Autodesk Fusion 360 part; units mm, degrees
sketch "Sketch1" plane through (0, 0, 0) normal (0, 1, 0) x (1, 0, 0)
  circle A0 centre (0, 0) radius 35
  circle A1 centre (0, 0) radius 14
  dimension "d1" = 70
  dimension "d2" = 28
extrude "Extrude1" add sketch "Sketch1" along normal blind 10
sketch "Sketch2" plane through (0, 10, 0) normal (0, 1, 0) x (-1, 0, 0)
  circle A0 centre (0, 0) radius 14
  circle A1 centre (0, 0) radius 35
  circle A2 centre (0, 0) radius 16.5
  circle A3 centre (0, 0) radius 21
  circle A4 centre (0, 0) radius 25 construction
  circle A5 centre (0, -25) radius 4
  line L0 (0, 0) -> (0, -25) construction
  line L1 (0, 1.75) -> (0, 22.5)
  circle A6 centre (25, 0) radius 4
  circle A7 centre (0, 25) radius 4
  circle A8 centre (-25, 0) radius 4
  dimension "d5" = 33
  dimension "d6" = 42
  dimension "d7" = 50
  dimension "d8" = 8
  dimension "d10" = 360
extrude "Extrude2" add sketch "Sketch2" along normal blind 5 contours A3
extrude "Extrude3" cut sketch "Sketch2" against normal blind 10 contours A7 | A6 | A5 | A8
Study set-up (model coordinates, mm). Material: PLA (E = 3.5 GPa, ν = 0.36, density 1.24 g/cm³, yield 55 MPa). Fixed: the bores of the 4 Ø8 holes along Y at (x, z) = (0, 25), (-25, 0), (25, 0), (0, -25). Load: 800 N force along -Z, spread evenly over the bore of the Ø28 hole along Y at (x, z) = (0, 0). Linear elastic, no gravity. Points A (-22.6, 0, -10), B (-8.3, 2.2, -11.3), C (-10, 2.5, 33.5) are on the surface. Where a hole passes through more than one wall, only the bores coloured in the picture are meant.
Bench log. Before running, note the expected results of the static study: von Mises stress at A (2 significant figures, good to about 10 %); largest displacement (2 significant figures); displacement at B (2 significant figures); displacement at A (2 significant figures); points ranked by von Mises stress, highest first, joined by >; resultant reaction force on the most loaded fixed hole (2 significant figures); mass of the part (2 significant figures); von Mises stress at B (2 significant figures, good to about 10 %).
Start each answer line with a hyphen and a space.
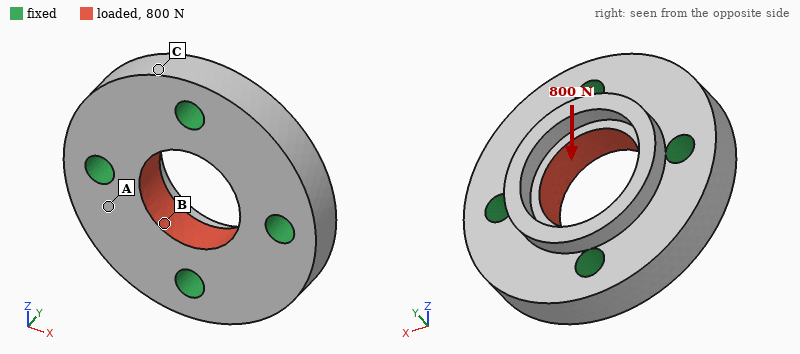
- 0.63 MPa
- 6.0 µm
- 5.3 µm
- 2.1 µm
- B > A > C
- 220 N
- 41 g
- 1.2 MPa
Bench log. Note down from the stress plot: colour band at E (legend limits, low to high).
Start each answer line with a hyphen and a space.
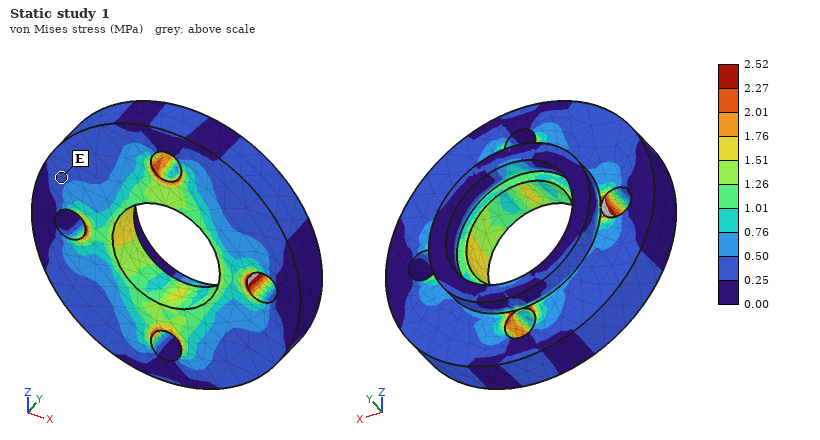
- 0.25 to 0.50 MPa
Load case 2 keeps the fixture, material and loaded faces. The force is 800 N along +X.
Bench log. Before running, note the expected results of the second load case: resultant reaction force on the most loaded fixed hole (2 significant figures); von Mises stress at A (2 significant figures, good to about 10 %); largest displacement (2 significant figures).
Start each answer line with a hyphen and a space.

- 220 N
- 0.63 MPa
- 6.0 µm
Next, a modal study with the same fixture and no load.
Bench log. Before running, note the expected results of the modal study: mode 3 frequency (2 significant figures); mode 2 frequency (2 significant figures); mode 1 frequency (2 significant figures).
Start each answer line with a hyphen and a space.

- 7900 Hz
- 7900 Hz
- 7500 Hz
